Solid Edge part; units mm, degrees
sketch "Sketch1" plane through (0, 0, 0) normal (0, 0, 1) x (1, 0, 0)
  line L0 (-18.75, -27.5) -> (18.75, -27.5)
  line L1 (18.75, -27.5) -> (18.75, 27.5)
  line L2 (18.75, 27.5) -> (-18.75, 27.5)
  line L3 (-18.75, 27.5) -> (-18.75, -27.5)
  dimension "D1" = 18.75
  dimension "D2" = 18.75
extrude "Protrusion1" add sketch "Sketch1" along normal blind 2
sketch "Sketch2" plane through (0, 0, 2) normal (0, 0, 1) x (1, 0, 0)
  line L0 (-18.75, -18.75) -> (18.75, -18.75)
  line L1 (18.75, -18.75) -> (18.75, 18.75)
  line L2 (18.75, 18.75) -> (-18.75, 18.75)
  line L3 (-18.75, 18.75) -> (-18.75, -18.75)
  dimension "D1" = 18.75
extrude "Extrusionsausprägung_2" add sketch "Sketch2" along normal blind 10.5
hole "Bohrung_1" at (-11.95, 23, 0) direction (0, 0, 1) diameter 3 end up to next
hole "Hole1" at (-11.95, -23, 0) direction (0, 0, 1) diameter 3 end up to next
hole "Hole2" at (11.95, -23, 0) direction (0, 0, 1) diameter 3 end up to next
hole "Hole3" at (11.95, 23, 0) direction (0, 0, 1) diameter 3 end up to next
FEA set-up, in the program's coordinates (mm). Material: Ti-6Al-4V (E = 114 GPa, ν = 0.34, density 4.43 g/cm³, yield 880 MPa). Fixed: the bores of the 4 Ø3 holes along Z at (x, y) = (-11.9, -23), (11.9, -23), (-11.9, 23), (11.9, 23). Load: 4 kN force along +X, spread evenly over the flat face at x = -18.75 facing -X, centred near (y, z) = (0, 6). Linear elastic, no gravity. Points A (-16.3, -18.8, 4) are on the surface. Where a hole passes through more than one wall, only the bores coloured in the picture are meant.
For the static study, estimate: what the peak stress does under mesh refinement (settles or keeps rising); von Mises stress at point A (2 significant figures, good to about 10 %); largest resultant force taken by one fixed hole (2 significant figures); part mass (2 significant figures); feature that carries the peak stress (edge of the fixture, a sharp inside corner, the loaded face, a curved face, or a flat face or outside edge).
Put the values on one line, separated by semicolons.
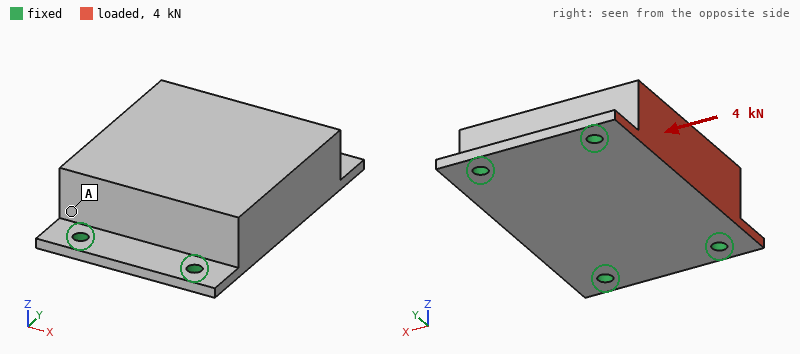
keeps rising; 24 MPa; 1.2 kN; 83 g; edge of the fixture
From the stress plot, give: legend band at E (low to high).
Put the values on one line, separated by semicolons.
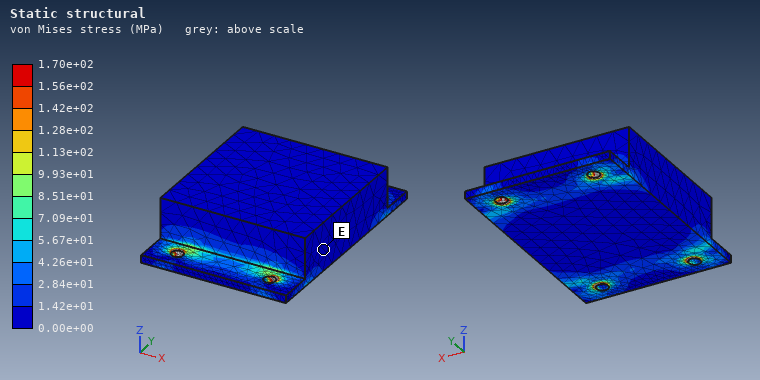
0.00e+00 to 1.42e+01 MPa
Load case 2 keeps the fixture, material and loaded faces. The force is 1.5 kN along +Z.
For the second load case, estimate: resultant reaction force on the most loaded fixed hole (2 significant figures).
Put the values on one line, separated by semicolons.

1.1 kN
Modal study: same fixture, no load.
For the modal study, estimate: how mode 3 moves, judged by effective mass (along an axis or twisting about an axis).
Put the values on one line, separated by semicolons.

along Y
